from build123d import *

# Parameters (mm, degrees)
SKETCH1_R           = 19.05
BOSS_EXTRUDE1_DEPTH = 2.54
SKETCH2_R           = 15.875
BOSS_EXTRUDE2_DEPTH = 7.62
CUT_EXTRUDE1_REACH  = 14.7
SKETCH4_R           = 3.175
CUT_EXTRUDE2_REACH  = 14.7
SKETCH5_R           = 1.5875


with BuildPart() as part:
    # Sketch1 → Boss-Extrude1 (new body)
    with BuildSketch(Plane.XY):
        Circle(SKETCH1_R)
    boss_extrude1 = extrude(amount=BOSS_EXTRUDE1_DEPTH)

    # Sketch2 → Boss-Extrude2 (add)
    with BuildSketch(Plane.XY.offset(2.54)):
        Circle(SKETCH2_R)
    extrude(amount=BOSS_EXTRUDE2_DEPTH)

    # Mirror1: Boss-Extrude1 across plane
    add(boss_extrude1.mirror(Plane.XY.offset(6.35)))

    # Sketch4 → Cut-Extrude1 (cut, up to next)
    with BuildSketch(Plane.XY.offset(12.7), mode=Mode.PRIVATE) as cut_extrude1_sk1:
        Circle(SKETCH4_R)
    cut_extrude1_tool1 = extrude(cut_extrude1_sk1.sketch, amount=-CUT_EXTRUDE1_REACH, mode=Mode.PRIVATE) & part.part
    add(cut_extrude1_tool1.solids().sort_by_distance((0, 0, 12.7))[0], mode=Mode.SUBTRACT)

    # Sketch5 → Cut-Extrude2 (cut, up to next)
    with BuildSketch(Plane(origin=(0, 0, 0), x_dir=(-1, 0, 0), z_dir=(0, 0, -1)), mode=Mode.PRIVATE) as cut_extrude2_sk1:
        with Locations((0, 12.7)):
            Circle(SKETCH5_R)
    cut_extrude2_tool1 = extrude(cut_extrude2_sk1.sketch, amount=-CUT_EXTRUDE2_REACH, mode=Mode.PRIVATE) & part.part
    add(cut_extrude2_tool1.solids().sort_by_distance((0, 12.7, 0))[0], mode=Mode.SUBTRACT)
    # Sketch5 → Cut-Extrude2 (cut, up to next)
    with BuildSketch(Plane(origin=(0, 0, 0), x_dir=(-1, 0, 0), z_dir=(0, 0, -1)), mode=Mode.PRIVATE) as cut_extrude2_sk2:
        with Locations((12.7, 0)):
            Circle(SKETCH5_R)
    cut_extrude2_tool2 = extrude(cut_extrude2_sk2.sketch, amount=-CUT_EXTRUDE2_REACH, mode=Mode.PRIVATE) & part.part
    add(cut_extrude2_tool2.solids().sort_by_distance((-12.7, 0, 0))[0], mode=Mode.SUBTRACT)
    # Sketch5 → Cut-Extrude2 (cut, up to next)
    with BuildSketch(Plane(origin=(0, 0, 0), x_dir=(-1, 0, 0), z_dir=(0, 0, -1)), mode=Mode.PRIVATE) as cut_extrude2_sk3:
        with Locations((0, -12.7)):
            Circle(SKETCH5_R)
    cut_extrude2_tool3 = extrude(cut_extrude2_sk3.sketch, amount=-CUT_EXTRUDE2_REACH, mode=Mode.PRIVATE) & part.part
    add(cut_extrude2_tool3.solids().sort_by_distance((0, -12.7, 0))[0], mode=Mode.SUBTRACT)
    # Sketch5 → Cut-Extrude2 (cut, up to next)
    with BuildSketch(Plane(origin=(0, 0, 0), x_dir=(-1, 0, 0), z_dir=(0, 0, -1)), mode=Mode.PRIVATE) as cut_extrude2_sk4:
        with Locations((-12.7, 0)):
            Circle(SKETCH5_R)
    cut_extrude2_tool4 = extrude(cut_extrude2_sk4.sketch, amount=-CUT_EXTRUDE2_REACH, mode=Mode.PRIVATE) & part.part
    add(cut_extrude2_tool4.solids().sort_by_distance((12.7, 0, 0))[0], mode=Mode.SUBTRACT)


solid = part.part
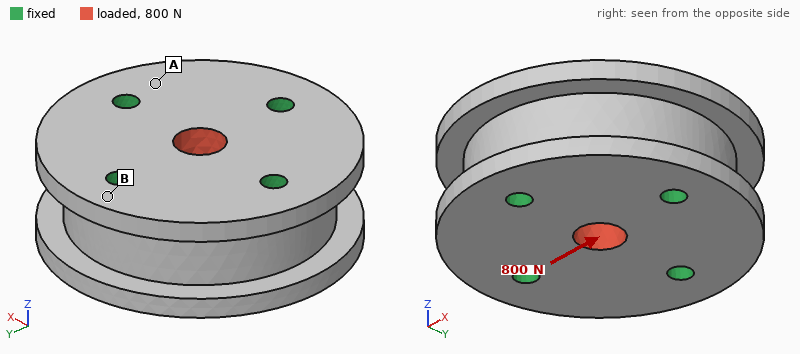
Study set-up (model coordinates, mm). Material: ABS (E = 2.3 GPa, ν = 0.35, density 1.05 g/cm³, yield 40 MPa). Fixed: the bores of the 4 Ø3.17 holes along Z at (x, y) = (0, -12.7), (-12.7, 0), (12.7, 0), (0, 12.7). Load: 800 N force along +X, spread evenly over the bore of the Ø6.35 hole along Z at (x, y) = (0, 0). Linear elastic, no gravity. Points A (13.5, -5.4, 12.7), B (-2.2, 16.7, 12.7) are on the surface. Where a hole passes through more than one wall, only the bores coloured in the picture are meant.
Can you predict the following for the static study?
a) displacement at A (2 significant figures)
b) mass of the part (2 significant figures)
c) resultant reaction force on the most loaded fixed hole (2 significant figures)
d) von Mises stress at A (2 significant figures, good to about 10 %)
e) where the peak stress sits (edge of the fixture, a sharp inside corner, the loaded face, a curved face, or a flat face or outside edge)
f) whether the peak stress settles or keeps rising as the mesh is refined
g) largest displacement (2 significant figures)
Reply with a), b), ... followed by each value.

a) 3.5 µm
b) 12 g
c) 270 N
d) 0.98 MPa
e) edge of the fixture
f) keeps rising
g) 13 µm
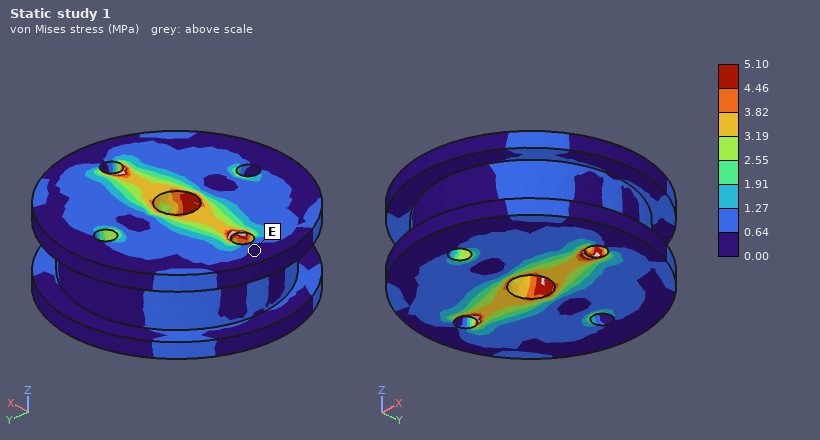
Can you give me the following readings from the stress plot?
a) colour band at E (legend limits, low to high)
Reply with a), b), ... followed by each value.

a) 0.00 to 0.64 MPa
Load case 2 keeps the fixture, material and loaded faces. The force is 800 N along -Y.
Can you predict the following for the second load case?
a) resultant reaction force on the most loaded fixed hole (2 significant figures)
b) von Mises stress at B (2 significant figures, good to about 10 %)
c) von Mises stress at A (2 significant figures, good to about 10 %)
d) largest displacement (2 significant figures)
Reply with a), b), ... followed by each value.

a) 270 N
b) 0.52 MPa
c) 0.74 MPa
d) 13 µm
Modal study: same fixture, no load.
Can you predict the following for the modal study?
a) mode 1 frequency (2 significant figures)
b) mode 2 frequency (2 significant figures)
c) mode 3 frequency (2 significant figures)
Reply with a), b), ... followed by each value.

a) 15 kHz
b) 16 kHz
c) 16 kHz
